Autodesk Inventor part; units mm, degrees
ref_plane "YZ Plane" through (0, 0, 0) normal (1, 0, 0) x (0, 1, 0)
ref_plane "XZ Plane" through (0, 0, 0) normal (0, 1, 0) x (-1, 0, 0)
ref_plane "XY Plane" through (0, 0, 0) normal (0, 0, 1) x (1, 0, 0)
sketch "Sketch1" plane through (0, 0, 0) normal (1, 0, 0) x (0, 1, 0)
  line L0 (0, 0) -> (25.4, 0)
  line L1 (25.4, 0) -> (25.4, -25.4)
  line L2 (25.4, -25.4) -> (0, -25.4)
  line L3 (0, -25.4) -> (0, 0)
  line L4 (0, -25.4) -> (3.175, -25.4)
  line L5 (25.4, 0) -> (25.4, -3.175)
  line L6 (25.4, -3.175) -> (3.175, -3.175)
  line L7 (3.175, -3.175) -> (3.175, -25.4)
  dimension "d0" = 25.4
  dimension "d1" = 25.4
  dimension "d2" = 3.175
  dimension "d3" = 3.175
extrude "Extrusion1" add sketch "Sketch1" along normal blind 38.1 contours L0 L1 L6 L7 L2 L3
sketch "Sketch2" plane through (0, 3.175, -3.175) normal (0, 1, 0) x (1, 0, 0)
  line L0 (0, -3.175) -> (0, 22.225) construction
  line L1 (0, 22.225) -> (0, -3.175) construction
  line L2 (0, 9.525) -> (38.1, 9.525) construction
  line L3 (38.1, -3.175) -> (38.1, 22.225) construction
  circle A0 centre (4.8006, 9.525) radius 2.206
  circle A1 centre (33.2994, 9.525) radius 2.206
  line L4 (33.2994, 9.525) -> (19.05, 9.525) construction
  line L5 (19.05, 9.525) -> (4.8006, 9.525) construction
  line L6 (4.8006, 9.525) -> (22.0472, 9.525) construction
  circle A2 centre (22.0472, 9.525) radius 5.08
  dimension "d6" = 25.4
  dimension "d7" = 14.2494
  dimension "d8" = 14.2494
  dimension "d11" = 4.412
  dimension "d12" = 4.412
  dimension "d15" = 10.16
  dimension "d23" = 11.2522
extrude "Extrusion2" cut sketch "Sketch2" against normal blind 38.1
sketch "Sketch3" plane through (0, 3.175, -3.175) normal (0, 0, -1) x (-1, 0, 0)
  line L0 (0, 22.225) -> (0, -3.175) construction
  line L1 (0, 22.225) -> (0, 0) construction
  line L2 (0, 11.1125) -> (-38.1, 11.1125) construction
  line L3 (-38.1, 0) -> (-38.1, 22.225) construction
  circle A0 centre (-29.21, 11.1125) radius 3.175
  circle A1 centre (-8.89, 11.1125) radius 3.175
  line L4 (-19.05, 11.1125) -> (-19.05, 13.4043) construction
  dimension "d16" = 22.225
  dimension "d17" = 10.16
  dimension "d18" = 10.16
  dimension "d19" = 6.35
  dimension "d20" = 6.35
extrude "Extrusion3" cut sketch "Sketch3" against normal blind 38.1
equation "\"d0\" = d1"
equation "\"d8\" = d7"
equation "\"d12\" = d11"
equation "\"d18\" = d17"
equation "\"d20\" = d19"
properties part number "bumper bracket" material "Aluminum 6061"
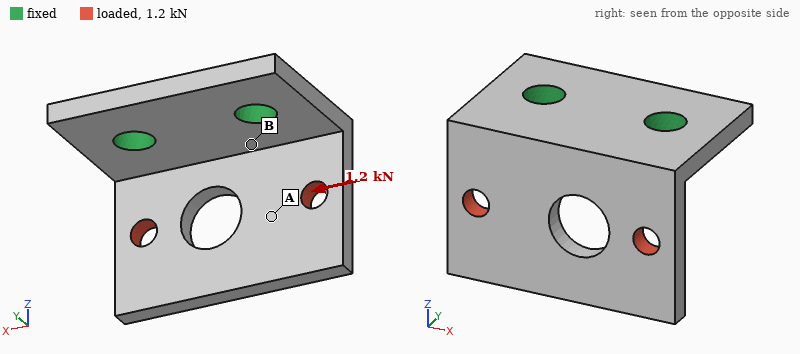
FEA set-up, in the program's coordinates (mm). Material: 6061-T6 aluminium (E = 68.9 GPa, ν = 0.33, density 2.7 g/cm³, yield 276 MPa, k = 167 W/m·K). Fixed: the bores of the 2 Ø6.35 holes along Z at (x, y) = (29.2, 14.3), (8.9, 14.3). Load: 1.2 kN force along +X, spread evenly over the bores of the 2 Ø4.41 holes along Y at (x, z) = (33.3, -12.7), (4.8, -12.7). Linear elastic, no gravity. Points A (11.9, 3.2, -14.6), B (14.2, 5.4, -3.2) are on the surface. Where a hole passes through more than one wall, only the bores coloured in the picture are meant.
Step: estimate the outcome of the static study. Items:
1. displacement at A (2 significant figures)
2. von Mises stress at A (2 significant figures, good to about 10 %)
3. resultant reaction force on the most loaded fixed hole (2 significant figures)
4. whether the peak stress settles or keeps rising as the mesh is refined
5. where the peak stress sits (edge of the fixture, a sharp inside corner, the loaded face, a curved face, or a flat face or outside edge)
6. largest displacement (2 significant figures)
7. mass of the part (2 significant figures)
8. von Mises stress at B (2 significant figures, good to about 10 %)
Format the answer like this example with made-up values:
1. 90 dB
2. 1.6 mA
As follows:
1. 0.069 mm
2. 31 MPa
3. 970 N
4. keeps rising
5. edge of the fixture
6. 0.14 mm
7. 14 g
8. 82 MPa
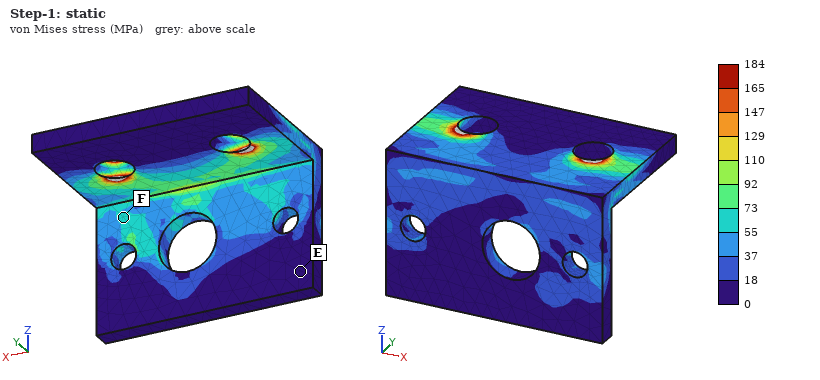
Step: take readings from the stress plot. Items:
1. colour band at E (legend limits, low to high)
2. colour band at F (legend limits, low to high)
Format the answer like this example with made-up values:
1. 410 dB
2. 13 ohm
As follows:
1. 0 to 18 MPa
2. 55 to 73 MPa
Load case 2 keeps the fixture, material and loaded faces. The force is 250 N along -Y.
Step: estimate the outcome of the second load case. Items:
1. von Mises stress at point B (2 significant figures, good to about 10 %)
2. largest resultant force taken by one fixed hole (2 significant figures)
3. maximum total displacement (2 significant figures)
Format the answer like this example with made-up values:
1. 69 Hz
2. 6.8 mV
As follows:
1. 38 MPa
2. 130 N
3. 0.14 mm
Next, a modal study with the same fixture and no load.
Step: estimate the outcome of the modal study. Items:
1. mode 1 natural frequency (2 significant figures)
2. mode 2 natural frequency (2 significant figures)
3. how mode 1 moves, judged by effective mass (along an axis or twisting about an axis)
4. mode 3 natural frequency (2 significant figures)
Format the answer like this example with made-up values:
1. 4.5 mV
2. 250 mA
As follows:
1. 2700 Hz
2. 5200 Hz
3. along Y
4. 7800 Hz
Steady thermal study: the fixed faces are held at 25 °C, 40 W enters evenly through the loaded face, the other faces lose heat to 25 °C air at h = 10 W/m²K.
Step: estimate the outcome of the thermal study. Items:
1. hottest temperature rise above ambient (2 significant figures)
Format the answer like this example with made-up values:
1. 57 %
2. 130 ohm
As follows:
1. 57 K
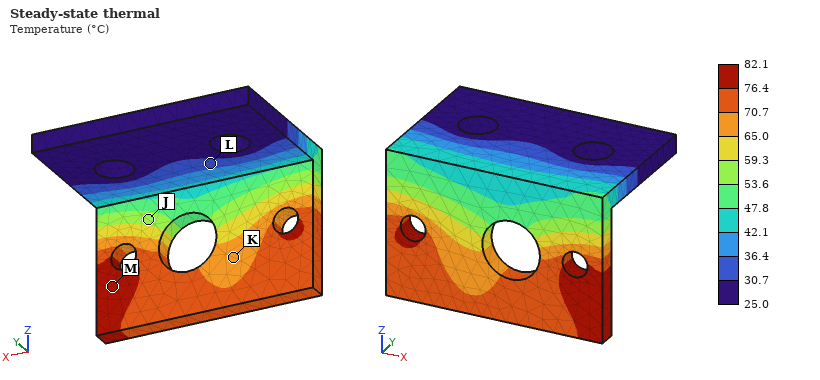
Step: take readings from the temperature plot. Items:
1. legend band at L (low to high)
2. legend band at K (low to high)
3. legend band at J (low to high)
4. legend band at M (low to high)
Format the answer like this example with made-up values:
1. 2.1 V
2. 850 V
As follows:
1. 30.7 to 36.4 °C
2. 65.0 to 70.7 °C
3. 53.6 to 59.3 °C
4. 76.4 to 82.1 °C
